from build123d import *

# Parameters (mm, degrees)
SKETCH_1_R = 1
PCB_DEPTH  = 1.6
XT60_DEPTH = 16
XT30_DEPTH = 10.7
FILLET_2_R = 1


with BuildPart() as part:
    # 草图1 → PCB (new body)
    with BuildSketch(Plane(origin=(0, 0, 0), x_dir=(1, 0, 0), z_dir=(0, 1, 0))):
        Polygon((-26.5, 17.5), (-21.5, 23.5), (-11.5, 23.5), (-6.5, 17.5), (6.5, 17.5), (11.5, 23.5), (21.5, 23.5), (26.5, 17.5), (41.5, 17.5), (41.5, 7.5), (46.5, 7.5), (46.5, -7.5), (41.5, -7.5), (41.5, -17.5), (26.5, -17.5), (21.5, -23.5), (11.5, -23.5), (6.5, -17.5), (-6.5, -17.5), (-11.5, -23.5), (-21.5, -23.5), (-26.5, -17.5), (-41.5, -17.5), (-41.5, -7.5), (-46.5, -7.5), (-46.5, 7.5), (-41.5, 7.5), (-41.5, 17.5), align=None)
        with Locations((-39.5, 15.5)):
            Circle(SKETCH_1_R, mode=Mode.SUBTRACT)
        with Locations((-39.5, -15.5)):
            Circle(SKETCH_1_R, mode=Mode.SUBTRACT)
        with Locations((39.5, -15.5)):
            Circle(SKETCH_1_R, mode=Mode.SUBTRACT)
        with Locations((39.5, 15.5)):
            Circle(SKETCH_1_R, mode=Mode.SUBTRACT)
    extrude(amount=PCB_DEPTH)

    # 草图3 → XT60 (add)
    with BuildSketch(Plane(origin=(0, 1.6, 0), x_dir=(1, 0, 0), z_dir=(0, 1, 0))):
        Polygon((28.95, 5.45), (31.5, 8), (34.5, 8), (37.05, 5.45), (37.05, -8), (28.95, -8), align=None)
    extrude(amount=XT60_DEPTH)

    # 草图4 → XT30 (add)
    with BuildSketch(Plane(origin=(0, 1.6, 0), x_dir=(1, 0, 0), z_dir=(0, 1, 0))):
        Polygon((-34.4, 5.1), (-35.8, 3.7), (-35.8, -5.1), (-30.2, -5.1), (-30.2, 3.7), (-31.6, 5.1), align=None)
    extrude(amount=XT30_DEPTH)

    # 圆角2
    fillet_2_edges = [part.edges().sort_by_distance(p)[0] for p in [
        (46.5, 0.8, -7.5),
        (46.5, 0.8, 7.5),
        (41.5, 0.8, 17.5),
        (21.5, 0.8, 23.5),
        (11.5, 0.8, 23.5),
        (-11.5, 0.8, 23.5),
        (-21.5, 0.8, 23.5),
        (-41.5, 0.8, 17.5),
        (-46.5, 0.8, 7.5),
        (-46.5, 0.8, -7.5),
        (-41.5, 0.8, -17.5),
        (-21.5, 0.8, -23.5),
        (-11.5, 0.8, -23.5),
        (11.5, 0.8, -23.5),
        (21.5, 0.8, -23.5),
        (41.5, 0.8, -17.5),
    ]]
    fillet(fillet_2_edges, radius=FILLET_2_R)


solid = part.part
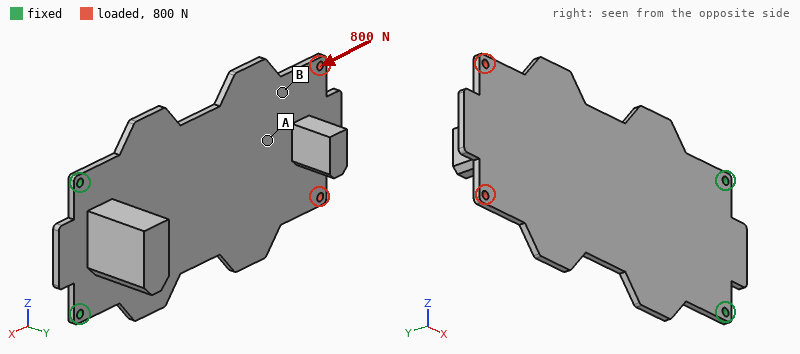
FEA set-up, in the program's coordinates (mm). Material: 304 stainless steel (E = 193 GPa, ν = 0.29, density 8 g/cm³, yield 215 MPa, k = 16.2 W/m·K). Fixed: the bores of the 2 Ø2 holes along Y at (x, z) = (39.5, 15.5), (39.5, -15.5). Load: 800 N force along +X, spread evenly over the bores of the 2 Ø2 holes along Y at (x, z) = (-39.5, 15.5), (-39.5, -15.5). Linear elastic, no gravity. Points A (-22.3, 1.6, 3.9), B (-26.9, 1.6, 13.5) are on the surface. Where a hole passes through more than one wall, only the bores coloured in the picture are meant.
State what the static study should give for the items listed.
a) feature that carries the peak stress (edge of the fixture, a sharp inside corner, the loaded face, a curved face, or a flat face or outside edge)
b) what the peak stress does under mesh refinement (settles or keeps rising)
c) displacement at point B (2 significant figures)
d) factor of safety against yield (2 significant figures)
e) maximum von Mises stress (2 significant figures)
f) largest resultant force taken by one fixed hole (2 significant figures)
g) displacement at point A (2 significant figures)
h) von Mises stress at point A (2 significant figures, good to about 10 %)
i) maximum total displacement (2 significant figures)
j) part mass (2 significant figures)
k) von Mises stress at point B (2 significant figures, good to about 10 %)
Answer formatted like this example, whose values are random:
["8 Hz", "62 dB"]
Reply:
["the loaded face", "settles", "6.3 µm", "1.4", "150 MPa", "420 N", "5.7 µm", "9.8 MPa", "10 µm", "64 g", "20 MPa"]
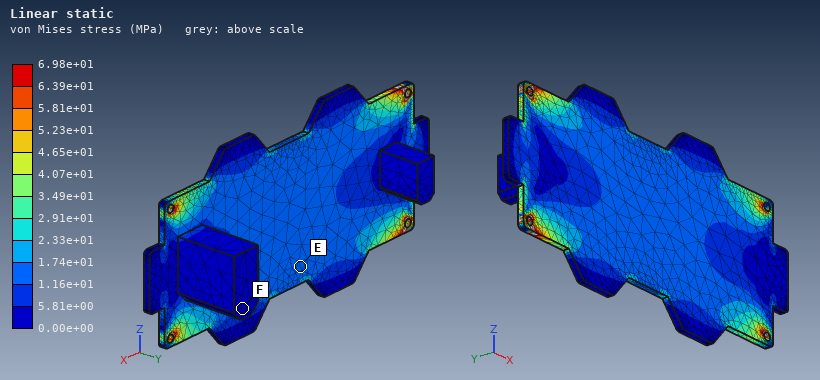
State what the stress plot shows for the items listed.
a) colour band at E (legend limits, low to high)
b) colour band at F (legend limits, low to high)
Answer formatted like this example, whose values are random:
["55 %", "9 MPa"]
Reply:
["1.16e+01 to 1.74e+01 MPa", "0.00e+00 to 5.81e+00 MPa"]
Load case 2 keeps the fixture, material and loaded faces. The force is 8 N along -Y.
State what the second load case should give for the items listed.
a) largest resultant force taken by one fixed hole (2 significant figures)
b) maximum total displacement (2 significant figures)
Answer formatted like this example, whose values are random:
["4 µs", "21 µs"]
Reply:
["4.4 N", "0.64 mm"]
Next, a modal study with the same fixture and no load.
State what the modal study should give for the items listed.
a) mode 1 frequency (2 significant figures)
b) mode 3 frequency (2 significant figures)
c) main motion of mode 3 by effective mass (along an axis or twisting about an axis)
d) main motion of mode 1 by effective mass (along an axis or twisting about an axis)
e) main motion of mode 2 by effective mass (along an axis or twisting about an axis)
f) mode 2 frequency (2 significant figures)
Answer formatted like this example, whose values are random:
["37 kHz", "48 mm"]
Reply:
["150 Hz", "950 Hz", "along Y", "along Y", "twisting about X", "830 Hz"]
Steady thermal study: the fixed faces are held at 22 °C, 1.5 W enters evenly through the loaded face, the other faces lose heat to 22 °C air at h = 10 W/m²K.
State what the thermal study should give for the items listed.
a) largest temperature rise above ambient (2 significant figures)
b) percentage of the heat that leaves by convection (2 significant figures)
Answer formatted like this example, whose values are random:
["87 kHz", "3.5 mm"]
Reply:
["67 K", "87 %"]
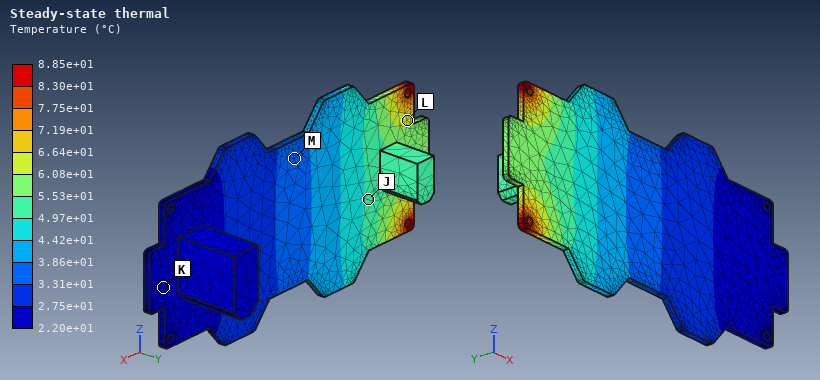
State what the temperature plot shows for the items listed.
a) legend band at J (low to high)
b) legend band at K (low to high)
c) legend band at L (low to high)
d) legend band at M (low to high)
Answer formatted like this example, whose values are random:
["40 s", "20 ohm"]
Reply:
["4.97e+01 to 5.53e+01 °C", "2.20e+01 to 2.75e+01 °C", "6.08e+01 to 6.64e+01 °C", "3.31e+01 to 3.86e+01 °C"]
